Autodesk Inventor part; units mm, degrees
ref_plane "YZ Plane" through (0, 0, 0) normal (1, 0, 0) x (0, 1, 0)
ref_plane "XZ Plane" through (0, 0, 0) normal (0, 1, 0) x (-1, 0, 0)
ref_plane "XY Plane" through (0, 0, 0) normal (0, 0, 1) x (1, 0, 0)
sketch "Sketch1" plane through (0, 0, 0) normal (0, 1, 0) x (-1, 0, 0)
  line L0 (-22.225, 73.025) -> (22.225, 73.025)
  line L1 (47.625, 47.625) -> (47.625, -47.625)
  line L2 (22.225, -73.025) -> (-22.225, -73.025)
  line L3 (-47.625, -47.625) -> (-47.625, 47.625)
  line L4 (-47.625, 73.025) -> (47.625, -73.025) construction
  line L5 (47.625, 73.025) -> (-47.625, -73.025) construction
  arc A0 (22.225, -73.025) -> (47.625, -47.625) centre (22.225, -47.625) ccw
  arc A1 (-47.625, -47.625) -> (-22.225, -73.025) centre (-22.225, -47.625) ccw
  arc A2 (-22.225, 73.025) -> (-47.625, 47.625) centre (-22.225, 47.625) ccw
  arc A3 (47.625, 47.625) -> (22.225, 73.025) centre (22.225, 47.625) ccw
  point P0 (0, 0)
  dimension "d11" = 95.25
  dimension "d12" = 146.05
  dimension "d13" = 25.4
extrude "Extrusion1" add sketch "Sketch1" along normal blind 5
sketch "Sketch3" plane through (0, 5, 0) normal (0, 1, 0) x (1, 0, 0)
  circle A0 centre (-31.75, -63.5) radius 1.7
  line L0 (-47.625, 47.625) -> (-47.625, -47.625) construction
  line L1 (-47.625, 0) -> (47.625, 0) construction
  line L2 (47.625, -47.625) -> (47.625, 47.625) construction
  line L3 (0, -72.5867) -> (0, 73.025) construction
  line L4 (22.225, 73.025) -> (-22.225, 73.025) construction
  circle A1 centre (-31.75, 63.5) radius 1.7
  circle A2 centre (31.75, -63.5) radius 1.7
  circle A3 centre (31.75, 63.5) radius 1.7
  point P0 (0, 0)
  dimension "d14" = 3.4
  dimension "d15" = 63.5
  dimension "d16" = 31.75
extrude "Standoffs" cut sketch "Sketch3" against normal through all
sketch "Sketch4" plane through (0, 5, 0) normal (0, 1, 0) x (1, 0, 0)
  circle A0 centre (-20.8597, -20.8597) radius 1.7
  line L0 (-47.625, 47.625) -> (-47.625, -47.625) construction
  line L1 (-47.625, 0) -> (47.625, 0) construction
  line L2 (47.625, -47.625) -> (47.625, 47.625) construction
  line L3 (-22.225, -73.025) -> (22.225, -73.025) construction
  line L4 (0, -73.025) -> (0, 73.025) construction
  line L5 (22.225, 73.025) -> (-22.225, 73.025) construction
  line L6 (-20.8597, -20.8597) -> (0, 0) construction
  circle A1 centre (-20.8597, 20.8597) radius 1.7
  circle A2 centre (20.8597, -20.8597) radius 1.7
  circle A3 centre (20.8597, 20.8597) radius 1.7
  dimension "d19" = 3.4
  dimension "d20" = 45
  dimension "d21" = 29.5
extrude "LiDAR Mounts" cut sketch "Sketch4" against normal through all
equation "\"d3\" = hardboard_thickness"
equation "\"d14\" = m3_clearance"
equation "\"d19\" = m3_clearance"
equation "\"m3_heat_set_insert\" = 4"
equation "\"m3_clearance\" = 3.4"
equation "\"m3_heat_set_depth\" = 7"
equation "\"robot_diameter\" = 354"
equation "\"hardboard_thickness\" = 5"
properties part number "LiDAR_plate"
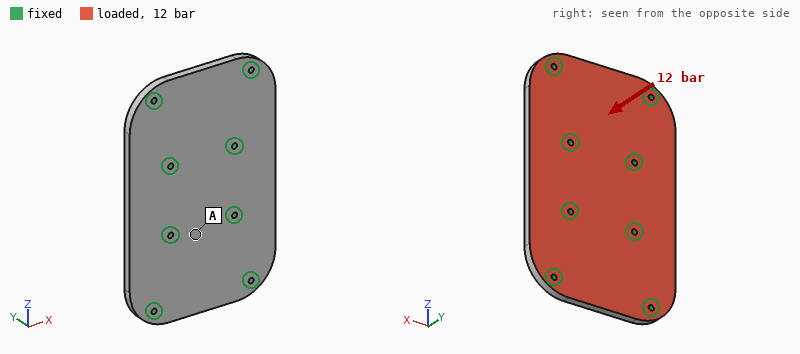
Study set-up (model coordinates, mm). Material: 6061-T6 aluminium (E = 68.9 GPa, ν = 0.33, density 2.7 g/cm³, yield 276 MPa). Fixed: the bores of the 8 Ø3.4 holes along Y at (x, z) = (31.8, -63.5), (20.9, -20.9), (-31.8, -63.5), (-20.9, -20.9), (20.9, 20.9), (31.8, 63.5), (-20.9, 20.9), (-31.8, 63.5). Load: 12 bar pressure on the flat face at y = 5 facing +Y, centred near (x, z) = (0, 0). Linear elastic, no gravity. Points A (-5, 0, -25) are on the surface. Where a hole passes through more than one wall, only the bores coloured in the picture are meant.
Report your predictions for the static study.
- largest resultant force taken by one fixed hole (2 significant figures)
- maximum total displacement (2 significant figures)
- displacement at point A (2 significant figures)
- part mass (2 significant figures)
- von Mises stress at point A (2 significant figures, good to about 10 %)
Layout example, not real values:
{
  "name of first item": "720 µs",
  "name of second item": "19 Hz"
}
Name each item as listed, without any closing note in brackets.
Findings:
{
  "largest resultant force taken by one fixed hole": "2.5 kN",
  "maximum total displacement": "0.13 mm",
  "displacement at point A": "0.020 mm",
  "part mass": "180 g",
  "von Mises stress at point A": "25 MPa"
}
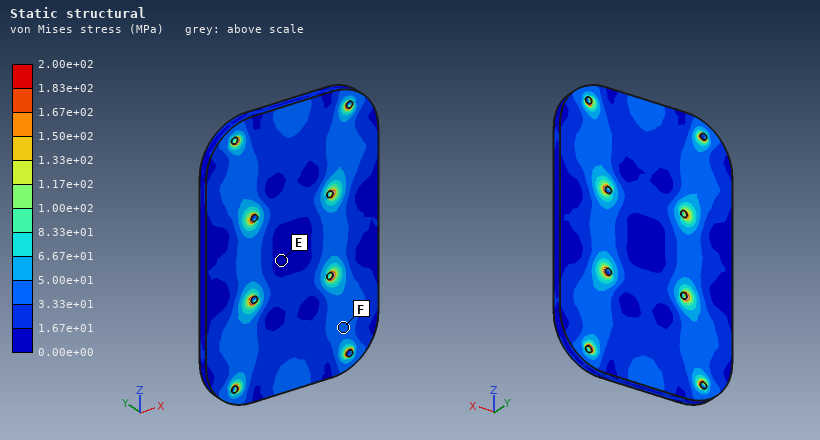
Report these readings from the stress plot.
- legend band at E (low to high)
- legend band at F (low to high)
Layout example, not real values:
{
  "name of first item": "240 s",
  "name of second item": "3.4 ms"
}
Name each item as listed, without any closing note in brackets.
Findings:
{
  "legend band at E": "0.00e+00 to 1.67e+01 MPa",
  "legend band at F": "3.33e+01 to 5.00e+01 MPa"
}
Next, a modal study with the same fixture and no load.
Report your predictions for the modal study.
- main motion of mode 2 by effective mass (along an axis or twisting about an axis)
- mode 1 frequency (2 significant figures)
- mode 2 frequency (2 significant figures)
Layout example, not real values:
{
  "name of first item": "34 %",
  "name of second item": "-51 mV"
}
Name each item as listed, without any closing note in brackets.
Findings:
{
  "main motion of mode 2 by effective mass": "twisting about Z",
  "mode 1 frequency": "4900 Hz",
  "mode 2 frequency": "5200 Hz"
}
